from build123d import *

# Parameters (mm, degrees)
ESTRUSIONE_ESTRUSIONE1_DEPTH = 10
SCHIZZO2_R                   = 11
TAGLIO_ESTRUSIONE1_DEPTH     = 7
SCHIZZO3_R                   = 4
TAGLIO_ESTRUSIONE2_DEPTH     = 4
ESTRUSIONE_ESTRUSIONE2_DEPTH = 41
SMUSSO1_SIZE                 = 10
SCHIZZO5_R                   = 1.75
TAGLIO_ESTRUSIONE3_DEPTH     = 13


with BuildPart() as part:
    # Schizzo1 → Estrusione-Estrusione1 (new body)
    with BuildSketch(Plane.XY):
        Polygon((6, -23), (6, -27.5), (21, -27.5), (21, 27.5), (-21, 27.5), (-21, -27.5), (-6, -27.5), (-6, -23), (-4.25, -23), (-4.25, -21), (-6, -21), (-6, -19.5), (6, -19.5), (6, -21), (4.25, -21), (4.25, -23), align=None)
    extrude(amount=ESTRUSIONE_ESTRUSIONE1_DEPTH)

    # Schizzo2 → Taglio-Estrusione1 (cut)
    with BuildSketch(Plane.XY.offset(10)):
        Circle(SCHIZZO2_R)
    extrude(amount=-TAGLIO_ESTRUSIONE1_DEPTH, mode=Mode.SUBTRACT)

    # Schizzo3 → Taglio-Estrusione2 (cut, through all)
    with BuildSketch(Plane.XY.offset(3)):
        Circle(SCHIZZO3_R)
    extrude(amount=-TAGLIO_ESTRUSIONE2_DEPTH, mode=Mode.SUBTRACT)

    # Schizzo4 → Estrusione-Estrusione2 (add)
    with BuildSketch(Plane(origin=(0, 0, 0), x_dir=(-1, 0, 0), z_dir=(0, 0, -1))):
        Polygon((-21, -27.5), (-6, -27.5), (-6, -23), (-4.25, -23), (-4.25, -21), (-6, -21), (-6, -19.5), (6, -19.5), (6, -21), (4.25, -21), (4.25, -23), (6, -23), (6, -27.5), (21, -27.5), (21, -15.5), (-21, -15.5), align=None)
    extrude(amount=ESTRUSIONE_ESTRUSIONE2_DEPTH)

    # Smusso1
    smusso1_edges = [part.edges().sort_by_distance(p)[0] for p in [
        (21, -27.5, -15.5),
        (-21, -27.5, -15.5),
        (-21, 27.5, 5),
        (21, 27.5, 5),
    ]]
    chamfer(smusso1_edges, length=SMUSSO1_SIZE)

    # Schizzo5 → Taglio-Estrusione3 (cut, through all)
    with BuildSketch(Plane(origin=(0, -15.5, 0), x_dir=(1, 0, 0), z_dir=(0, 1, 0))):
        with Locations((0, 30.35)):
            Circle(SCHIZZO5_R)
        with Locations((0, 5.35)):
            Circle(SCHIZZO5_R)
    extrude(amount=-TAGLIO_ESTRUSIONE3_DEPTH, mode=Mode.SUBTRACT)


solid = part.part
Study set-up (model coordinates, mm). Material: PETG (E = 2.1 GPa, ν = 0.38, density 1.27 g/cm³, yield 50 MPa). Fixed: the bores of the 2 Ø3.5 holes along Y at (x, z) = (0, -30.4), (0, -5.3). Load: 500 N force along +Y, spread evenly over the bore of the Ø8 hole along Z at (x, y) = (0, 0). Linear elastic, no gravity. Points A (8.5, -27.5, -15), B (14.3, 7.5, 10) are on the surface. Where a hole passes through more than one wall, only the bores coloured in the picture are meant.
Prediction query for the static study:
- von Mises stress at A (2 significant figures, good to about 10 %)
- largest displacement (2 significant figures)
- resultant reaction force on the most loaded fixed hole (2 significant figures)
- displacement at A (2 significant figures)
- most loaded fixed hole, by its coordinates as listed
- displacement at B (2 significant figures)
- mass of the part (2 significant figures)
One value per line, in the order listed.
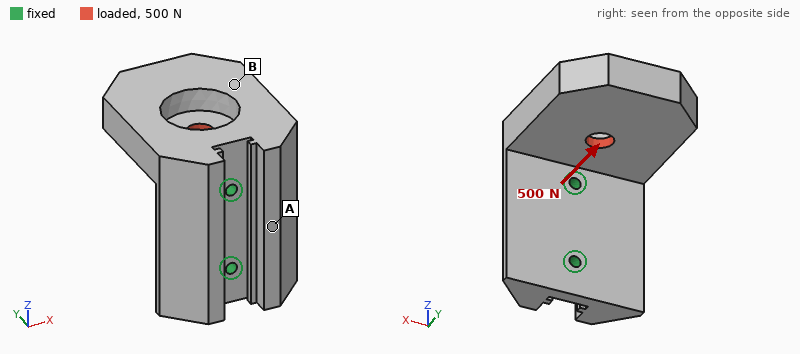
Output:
4.0 MPa
0.47 mm
590 N
0.074 mm
(0, -5.3)
0.36 mm
38 g
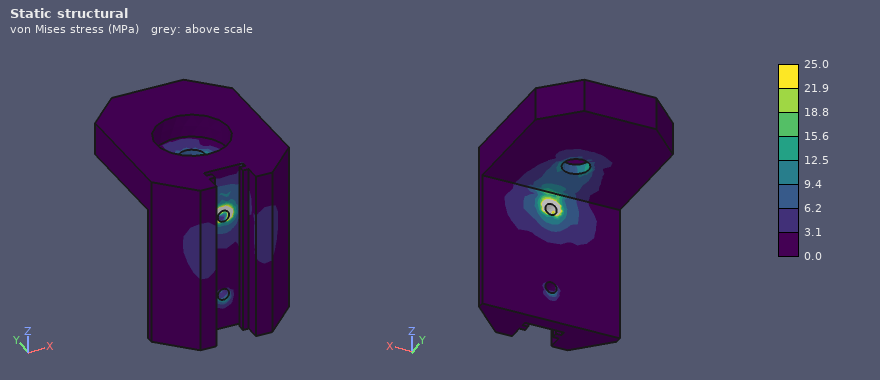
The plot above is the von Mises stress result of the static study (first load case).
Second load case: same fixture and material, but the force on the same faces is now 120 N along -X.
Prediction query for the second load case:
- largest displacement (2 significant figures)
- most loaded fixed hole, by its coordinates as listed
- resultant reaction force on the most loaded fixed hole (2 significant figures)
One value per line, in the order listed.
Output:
0.89 mm
(0, -5.3)
150 N
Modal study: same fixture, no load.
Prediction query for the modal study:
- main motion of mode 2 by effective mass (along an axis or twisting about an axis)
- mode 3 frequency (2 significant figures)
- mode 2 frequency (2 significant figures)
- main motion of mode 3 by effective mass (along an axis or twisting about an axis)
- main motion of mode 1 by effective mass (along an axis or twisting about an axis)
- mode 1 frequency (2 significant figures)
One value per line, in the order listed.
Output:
along Z
1600 Hz
530 Hz
twisting about Y
along X
400 Hz
